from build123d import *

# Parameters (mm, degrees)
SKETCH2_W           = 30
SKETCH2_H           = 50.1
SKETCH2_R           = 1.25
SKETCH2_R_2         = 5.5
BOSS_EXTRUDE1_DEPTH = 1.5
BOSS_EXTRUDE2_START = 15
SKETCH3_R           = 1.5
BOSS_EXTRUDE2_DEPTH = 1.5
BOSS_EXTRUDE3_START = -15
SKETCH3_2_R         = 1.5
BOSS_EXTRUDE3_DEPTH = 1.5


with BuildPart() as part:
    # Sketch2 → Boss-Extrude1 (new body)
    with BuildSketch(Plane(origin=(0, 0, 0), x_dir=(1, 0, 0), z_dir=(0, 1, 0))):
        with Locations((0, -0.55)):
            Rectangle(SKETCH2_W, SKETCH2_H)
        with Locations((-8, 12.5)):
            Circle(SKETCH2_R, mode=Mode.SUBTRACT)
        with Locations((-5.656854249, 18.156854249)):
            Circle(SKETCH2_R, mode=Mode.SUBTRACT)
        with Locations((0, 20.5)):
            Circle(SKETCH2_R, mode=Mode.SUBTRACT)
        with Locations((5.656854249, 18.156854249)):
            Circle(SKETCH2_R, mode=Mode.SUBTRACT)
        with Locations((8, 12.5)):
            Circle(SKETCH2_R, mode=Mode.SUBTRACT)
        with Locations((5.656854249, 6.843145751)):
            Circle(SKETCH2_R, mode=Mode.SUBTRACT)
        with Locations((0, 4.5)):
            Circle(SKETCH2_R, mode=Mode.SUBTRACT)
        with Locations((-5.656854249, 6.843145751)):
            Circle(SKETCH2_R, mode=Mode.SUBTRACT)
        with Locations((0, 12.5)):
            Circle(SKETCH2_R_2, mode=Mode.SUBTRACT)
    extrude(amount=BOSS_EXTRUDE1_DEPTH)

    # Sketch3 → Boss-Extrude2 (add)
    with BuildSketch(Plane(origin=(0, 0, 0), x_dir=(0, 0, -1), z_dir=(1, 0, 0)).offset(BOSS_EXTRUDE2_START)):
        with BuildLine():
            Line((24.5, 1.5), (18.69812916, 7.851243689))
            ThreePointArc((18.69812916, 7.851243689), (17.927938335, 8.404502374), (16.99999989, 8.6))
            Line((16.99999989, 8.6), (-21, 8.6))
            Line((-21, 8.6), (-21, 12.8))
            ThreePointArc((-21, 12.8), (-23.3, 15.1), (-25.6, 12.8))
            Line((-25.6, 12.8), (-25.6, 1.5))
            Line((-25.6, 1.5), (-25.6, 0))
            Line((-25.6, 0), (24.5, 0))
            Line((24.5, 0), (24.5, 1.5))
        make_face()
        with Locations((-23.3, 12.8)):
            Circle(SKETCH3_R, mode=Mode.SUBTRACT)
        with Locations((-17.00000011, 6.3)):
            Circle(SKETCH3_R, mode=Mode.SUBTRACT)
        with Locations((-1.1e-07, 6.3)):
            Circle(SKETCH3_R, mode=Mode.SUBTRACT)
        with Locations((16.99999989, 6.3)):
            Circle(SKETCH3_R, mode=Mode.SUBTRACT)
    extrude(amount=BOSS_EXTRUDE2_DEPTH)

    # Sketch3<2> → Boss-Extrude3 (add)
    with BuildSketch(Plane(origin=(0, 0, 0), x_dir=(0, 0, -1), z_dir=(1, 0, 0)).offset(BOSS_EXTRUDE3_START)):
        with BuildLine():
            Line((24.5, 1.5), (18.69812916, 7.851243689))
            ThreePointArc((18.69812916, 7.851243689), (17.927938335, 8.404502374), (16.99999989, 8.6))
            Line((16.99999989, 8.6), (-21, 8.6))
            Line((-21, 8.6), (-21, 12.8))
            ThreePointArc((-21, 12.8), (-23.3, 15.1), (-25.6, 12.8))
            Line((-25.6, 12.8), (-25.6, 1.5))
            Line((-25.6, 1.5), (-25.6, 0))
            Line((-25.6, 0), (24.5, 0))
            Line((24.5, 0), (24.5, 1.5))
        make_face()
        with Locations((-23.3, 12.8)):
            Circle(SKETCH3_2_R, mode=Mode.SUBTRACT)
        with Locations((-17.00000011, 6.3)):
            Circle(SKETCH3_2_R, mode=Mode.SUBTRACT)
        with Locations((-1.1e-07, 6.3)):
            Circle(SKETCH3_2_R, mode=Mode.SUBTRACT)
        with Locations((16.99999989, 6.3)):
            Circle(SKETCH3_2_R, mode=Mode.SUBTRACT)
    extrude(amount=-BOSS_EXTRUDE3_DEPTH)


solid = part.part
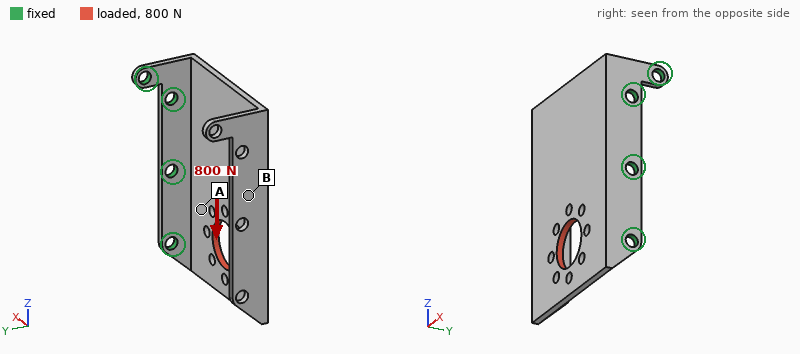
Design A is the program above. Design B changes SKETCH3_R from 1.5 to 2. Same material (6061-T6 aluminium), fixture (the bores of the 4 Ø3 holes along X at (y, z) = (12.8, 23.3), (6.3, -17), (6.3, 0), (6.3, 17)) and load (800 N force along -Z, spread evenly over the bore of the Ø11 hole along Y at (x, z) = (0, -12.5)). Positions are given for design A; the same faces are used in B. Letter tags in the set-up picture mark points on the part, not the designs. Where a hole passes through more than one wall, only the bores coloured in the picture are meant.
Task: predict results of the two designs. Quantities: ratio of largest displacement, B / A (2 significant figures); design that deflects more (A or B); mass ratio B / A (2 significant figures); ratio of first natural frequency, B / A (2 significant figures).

0.80
A
0.99
1.0
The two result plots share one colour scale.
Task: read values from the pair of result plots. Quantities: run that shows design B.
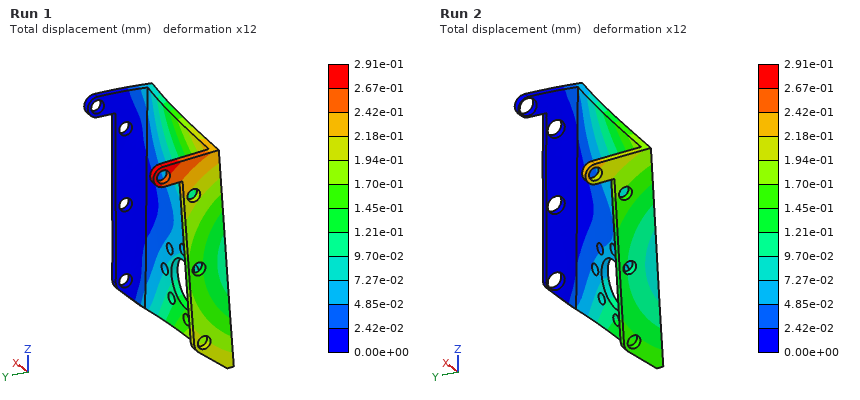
Run 2
